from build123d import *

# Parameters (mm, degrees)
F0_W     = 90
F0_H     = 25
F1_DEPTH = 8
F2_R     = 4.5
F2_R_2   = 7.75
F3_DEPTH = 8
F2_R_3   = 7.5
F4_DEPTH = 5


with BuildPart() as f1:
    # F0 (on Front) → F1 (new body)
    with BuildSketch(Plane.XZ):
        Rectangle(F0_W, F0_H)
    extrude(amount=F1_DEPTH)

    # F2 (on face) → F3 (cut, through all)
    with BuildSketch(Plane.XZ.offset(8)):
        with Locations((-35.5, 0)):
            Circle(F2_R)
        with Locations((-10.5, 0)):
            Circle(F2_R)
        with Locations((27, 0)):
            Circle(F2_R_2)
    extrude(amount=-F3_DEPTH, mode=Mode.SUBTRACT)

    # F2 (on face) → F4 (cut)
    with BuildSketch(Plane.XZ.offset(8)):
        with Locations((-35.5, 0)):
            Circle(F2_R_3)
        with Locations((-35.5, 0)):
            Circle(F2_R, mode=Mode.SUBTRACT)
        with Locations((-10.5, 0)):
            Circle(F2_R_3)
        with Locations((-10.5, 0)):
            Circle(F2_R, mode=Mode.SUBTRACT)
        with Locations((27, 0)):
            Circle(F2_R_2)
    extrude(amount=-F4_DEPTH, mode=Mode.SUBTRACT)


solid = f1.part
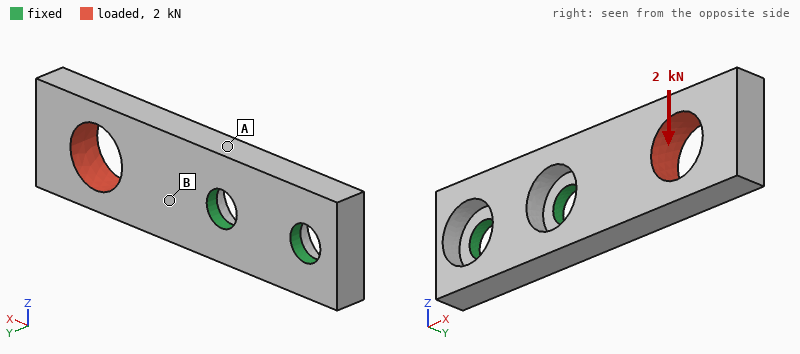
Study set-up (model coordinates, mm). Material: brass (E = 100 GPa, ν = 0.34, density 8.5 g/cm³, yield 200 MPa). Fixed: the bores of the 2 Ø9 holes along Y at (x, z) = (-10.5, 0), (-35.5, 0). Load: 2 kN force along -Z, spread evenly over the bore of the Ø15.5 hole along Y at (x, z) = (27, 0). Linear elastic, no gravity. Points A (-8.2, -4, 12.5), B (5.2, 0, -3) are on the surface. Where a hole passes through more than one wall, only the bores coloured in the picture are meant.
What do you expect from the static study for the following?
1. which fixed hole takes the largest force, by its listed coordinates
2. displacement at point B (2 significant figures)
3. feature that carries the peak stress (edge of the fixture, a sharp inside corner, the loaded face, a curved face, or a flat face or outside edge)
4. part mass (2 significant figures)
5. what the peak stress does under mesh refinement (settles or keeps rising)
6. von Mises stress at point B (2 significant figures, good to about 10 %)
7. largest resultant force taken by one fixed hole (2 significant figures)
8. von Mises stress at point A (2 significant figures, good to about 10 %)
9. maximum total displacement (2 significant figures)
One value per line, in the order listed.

(-10.5, 0)
0.025 mm
edge of the fixture
120 g
keeps rising
25 MPa
3.6 kN
82 MPa
0.14 mm
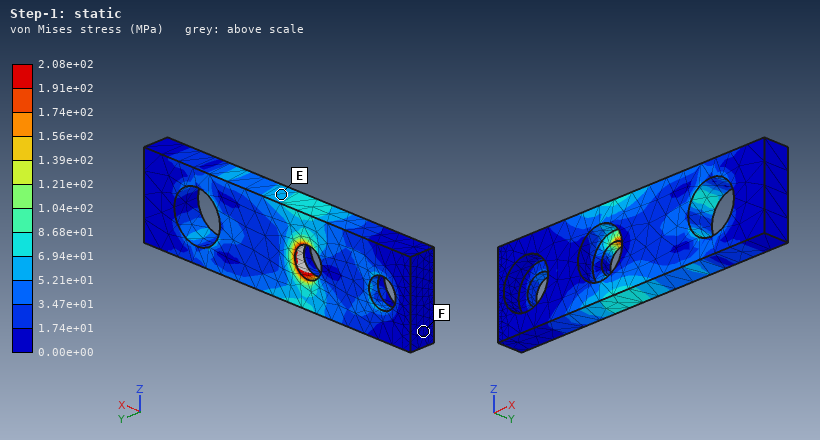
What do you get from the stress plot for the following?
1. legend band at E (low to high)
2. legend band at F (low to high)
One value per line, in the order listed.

5.21e+01 to 6.94e+01 MPa
0.00e+00 to 1.74e+01 MPa
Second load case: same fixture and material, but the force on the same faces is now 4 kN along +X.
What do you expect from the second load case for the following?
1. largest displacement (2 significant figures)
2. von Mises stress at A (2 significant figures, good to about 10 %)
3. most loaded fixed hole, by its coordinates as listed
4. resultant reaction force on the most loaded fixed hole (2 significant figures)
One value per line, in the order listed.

62 µm
18 MPa
(-10.5, 0)
3.0 kN
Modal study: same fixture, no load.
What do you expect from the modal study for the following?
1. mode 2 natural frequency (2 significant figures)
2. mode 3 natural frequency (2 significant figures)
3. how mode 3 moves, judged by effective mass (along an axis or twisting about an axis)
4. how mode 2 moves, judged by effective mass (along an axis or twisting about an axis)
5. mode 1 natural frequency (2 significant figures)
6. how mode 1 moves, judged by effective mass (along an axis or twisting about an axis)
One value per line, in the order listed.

3100 Hz
4200 Hz
twisting about X
along Z
1300 Hz
along Y
